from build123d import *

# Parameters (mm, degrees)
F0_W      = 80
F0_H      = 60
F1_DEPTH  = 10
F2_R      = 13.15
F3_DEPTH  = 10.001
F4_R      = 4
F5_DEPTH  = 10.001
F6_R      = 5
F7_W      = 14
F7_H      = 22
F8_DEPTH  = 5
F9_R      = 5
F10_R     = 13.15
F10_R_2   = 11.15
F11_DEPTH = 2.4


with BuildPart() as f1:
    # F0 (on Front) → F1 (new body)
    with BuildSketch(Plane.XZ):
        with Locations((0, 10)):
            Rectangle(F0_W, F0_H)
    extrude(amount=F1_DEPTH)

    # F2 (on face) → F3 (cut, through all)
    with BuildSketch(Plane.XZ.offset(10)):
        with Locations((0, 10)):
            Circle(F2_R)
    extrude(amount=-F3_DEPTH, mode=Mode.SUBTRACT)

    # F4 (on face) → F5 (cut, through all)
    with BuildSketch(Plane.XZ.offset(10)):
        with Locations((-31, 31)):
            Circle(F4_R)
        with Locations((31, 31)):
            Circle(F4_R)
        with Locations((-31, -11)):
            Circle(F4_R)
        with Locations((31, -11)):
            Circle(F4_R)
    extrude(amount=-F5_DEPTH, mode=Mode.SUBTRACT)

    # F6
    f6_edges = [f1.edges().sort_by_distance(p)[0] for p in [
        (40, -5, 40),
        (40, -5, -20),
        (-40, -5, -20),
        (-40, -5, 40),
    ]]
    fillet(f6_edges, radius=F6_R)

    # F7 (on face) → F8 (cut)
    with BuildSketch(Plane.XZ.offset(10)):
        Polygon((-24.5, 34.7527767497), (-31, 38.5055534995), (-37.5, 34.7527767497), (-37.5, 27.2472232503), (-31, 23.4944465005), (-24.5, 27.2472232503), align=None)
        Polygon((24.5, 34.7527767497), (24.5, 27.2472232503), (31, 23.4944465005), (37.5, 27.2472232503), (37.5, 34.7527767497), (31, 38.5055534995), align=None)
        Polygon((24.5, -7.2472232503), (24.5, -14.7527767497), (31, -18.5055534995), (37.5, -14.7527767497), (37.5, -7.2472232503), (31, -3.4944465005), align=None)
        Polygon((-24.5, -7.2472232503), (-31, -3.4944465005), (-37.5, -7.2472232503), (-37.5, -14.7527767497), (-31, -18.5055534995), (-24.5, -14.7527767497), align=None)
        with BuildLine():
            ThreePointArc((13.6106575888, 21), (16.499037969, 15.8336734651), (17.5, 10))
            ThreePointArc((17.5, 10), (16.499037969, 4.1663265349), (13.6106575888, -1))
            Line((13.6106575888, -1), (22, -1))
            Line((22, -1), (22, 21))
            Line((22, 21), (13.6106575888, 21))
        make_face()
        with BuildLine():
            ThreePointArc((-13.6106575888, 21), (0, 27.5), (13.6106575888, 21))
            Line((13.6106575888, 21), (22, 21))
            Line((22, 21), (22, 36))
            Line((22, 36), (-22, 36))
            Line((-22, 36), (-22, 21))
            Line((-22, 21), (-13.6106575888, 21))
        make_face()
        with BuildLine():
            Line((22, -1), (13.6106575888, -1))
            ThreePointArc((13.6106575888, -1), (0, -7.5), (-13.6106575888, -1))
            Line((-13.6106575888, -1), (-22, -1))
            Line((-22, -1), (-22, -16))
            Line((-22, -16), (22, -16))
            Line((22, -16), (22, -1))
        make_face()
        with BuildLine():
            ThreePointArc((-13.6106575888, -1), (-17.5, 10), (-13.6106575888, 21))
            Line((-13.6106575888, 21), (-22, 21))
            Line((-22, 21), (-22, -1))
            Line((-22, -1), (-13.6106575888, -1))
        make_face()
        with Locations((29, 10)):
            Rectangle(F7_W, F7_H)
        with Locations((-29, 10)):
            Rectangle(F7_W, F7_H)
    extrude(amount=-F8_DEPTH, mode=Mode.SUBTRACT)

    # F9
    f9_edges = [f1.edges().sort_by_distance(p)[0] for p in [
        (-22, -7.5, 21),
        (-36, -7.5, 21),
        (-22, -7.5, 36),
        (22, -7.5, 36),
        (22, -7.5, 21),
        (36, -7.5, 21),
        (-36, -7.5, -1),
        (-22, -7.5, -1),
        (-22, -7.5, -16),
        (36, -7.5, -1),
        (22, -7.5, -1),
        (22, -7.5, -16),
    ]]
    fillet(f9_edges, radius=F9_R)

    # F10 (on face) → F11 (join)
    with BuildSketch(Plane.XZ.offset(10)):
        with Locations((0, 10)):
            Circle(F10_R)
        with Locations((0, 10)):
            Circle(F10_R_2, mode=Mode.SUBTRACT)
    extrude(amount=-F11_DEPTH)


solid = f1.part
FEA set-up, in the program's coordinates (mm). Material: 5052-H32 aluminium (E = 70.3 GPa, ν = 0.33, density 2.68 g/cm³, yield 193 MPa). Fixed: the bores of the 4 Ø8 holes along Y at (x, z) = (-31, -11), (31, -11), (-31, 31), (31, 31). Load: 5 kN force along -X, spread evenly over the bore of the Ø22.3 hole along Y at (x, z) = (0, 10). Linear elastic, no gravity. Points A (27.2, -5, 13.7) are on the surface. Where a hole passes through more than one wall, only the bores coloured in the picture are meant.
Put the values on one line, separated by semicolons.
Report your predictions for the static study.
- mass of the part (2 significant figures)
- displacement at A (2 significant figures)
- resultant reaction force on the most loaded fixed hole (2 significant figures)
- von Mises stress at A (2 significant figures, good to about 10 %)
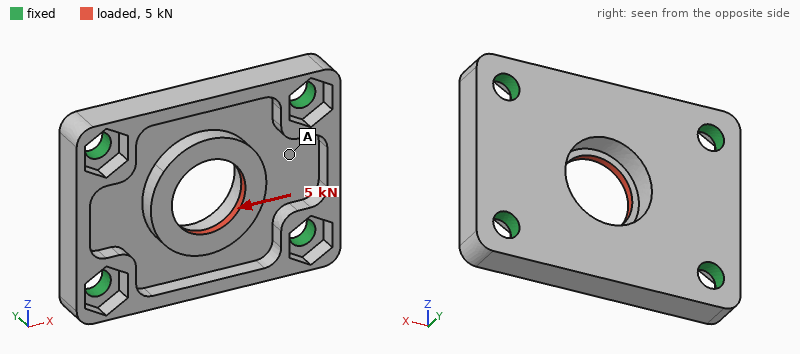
78 g; 5.5 µm; 1.3 kN; 10 MPa
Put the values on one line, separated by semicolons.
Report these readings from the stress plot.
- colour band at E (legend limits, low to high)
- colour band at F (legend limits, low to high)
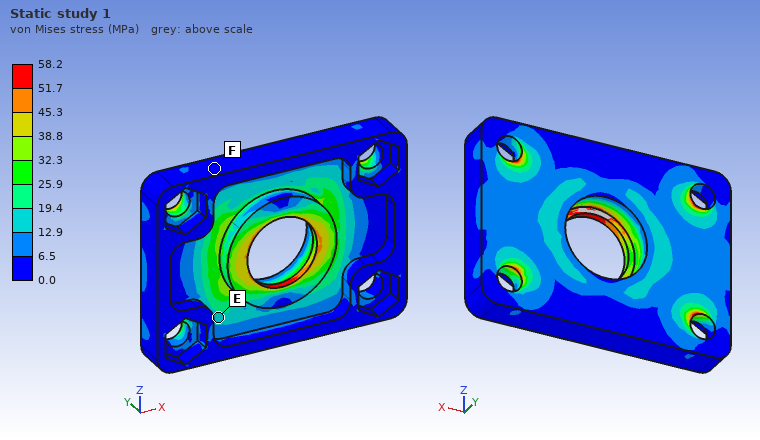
12.9 to 19.4 MPa; 0.0 to 6.5 MPa
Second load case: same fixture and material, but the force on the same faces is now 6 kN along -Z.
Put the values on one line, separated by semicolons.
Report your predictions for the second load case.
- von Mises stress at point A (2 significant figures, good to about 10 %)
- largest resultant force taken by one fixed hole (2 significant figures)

24 MPa; 1.8 kN
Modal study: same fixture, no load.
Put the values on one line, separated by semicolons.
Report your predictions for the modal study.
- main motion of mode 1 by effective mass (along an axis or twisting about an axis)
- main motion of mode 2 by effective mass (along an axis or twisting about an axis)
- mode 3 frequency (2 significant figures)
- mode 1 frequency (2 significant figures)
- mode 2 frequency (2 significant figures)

along Y; twisting about X; 14 kHz; 9100 Hz; 11 kHz
